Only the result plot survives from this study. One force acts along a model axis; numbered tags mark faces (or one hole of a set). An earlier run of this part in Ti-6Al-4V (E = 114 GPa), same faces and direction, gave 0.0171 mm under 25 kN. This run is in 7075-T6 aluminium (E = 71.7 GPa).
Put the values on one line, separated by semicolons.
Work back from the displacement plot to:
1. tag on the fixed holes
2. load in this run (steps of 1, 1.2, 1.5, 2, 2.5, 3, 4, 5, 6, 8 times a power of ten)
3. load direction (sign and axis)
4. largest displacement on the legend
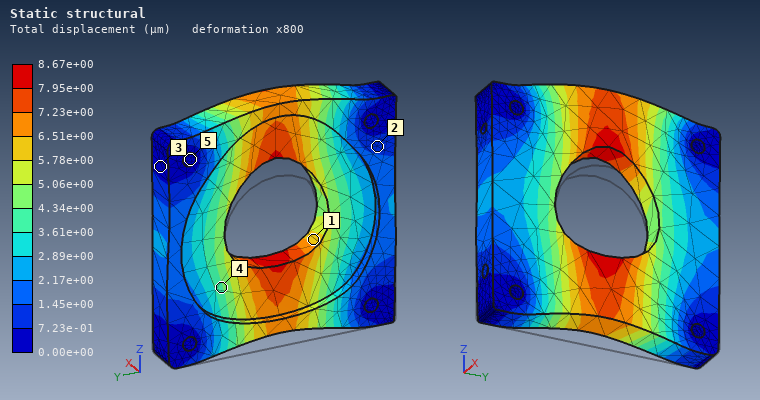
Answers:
5; 8 kN; +Z; 8.67e+00 µm
